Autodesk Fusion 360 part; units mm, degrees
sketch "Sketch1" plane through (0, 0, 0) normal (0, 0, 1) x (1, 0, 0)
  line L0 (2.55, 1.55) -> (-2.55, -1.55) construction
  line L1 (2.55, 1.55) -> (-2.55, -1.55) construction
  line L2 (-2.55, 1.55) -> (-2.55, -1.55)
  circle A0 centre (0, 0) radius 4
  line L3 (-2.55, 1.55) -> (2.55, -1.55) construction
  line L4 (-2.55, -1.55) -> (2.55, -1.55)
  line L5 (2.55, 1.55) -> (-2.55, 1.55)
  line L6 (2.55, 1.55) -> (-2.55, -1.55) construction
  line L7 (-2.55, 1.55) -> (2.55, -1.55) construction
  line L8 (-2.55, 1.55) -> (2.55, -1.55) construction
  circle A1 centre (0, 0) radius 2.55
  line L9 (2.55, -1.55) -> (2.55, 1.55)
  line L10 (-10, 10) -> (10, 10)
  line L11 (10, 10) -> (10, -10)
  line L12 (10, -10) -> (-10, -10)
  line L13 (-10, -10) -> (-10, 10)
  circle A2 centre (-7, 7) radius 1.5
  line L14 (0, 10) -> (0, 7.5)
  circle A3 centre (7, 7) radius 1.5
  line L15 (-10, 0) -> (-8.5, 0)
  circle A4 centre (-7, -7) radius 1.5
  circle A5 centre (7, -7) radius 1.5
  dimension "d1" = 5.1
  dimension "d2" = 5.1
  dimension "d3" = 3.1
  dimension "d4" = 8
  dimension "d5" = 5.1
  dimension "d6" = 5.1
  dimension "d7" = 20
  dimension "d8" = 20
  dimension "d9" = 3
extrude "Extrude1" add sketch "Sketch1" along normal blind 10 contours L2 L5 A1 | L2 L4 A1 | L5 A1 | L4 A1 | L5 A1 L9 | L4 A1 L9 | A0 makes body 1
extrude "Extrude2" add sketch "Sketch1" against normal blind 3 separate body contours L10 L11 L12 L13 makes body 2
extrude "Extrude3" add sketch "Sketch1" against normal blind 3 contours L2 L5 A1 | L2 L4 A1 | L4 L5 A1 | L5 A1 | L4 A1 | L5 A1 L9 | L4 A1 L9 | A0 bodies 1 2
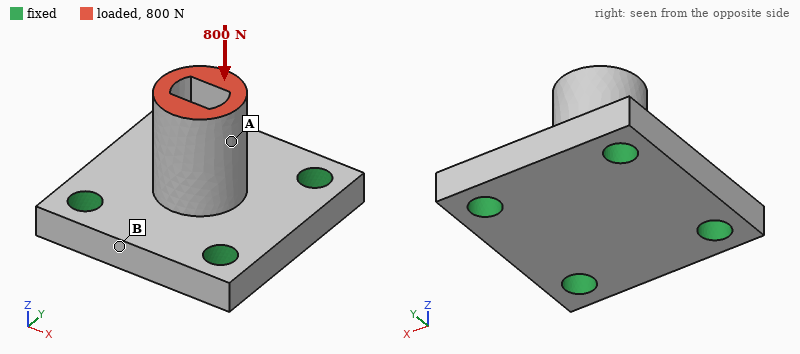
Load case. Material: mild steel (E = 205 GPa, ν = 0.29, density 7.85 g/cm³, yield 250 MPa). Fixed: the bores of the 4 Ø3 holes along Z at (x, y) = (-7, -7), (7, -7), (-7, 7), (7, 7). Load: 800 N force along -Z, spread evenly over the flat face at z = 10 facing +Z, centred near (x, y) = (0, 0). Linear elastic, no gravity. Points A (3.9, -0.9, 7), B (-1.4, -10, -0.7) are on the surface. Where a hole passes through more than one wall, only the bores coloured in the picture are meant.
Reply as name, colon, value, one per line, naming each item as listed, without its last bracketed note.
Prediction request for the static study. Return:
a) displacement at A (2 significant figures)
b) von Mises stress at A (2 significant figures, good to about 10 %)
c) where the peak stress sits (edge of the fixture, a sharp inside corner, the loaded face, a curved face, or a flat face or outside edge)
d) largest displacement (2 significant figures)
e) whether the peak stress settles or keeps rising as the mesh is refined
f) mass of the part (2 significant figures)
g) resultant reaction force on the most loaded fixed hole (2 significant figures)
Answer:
displacement at A: 2.8 µm
von Mises stress at A: 23 MPa
where the peak stress sits: edge of the fixture
largest displacement: 3.1 µm
whether the peak stress settles or keeps rising as the mesh is refined: keeps rising
mass of the part: 12 g
resultant reaction force on the most loaded fixed hole: 200 N
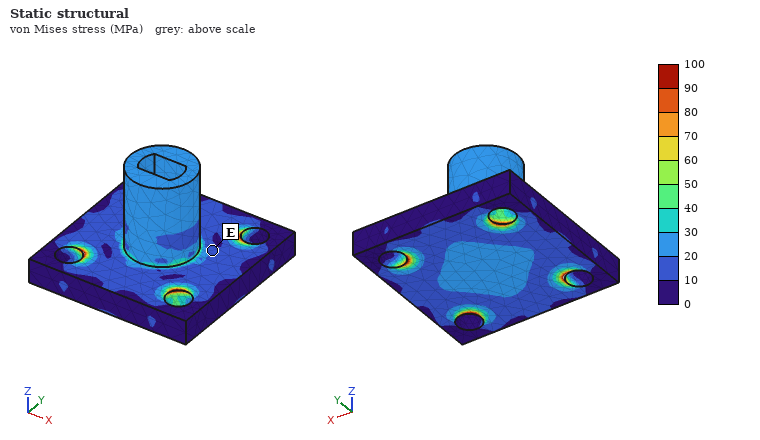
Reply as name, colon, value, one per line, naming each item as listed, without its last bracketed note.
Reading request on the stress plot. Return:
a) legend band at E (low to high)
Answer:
legend band at E: 10 to 20 MPa
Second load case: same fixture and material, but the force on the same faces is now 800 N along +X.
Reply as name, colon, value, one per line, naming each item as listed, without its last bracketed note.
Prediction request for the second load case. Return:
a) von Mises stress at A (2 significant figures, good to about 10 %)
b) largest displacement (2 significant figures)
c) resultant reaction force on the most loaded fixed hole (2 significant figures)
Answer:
von Mises stress at A: 65 MPa
largest displacement: 25 µm
resultant reaction force on the most loaded fixed hole: 460 N
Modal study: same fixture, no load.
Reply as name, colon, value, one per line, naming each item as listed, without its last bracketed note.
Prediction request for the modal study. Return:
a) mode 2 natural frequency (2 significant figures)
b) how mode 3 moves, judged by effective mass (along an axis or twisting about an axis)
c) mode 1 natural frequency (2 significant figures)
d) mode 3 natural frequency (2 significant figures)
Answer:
mode 2 natural frequency: 29 kHz
how mode 3 moves, judged by effective mass: along Z
mode 1 natural frequency: 29 kHz
mode 3 natural frequency: 42 kHz
